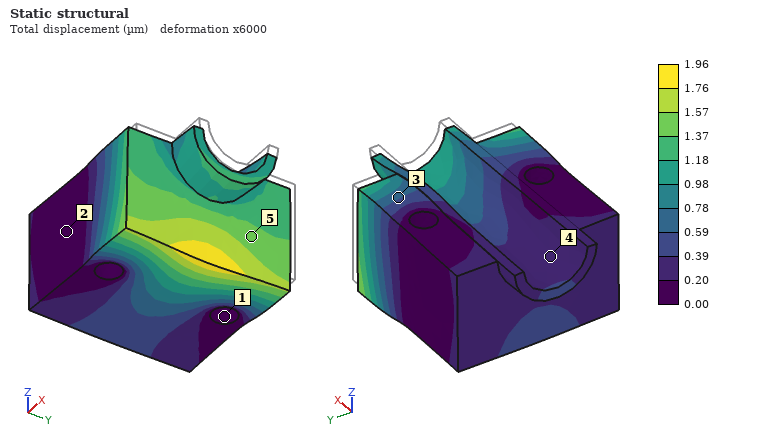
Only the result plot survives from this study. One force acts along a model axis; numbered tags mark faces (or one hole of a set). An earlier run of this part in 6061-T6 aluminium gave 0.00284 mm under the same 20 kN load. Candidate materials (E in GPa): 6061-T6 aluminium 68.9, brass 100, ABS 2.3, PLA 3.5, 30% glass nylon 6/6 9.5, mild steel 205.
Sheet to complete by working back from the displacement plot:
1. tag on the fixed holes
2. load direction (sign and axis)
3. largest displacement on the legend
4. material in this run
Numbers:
1
-X
1.96 µm
brass
